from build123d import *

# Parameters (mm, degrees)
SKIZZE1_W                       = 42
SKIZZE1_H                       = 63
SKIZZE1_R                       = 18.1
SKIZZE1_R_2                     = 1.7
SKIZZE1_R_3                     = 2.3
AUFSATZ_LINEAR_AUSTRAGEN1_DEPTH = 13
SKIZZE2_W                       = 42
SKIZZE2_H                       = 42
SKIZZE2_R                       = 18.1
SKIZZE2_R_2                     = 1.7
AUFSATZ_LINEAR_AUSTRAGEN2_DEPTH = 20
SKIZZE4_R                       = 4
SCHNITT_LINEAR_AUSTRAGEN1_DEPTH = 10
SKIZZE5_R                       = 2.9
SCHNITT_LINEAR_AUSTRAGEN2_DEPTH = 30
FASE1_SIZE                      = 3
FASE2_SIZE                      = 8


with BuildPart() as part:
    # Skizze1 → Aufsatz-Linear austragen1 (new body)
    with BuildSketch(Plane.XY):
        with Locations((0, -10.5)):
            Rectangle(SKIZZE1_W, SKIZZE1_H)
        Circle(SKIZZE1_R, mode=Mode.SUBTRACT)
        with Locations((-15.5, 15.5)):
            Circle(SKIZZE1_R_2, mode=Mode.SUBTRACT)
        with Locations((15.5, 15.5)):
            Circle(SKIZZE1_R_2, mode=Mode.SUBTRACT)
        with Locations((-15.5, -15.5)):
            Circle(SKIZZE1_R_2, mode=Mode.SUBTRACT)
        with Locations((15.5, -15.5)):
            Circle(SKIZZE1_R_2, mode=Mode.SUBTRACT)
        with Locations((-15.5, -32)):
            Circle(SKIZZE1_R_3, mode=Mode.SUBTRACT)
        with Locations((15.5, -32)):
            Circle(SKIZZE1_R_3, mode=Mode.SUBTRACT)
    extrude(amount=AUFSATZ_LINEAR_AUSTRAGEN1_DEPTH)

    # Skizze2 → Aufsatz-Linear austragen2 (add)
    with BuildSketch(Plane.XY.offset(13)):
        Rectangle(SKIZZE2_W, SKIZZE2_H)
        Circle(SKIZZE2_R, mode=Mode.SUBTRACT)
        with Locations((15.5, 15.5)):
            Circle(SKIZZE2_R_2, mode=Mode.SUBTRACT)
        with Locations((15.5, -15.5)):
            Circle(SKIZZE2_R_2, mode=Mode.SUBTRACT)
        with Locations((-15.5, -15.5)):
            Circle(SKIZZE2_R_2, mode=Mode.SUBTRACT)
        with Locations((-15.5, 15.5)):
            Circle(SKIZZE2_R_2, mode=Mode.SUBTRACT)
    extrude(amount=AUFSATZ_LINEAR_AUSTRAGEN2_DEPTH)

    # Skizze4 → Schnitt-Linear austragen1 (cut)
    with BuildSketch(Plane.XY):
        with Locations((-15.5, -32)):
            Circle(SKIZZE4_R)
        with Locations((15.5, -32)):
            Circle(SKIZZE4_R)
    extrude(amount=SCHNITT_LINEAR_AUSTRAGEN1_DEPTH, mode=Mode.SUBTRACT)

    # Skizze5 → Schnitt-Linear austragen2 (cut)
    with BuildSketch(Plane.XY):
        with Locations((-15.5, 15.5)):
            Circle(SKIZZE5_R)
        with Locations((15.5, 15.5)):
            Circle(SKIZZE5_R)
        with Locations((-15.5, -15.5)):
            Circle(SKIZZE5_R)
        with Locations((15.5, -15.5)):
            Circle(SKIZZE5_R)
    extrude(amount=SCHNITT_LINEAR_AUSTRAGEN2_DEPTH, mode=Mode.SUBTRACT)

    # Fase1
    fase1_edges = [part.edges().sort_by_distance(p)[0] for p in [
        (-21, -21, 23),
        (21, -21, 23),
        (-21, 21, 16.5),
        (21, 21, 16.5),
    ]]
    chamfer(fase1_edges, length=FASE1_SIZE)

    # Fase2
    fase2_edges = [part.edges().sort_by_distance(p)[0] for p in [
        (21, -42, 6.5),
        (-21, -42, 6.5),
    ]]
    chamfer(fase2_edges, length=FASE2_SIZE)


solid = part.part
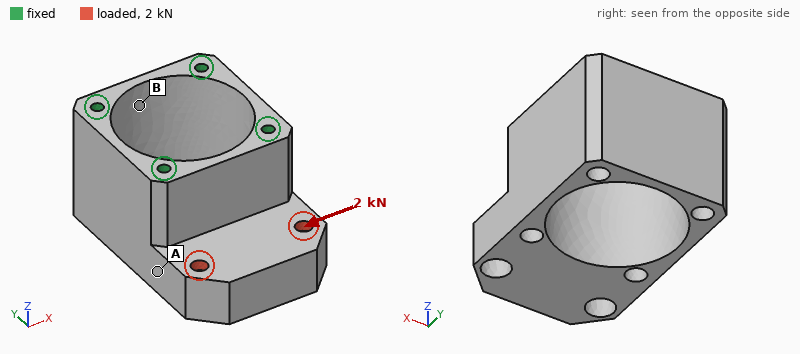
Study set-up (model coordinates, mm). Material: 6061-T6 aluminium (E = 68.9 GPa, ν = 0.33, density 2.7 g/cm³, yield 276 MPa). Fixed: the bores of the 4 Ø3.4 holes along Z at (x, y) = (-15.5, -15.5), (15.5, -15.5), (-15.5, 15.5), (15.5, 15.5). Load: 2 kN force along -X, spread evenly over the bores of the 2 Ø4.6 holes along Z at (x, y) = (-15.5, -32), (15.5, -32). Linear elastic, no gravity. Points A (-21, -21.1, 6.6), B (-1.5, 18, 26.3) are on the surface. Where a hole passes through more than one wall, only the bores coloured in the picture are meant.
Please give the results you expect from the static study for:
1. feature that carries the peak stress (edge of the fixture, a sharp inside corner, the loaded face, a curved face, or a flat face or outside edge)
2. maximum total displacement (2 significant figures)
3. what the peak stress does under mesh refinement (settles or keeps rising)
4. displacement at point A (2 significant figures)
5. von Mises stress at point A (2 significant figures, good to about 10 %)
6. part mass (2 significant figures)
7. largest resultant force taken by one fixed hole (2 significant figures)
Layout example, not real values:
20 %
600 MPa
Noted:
edge of the fixture
31 µm
keeps rising
20 µm
15 MPa
81 g
1.3 kN
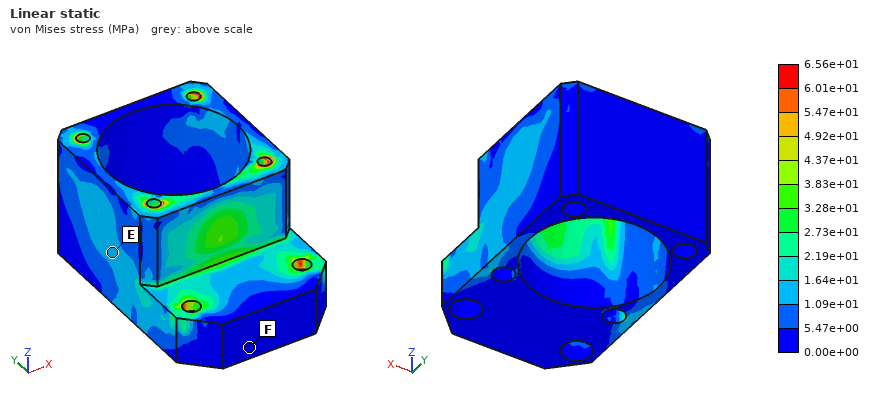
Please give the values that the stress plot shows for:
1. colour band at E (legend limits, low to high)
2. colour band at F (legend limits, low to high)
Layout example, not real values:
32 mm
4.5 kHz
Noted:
1.09e+01 to 1.64e+01 MPa
0.00e+00 to 5.47e+00 MPa
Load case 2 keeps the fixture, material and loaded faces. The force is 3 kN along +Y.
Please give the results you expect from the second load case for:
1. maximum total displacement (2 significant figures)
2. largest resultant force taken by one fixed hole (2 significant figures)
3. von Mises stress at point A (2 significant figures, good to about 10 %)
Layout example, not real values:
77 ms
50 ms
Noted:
30 µm
1.3 kN
20 MPa
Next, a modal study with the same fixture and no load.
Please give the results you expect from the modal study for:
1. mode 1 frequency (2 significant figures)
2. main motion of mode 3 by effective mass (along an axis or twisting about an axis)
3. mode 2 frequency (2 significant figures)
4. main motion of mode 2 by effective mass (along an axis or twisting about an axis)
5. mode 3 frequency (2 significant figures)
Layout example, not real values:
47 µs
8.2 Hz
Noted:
6000 Hz
along Y
7200 Hz
along X
10000 Hz
